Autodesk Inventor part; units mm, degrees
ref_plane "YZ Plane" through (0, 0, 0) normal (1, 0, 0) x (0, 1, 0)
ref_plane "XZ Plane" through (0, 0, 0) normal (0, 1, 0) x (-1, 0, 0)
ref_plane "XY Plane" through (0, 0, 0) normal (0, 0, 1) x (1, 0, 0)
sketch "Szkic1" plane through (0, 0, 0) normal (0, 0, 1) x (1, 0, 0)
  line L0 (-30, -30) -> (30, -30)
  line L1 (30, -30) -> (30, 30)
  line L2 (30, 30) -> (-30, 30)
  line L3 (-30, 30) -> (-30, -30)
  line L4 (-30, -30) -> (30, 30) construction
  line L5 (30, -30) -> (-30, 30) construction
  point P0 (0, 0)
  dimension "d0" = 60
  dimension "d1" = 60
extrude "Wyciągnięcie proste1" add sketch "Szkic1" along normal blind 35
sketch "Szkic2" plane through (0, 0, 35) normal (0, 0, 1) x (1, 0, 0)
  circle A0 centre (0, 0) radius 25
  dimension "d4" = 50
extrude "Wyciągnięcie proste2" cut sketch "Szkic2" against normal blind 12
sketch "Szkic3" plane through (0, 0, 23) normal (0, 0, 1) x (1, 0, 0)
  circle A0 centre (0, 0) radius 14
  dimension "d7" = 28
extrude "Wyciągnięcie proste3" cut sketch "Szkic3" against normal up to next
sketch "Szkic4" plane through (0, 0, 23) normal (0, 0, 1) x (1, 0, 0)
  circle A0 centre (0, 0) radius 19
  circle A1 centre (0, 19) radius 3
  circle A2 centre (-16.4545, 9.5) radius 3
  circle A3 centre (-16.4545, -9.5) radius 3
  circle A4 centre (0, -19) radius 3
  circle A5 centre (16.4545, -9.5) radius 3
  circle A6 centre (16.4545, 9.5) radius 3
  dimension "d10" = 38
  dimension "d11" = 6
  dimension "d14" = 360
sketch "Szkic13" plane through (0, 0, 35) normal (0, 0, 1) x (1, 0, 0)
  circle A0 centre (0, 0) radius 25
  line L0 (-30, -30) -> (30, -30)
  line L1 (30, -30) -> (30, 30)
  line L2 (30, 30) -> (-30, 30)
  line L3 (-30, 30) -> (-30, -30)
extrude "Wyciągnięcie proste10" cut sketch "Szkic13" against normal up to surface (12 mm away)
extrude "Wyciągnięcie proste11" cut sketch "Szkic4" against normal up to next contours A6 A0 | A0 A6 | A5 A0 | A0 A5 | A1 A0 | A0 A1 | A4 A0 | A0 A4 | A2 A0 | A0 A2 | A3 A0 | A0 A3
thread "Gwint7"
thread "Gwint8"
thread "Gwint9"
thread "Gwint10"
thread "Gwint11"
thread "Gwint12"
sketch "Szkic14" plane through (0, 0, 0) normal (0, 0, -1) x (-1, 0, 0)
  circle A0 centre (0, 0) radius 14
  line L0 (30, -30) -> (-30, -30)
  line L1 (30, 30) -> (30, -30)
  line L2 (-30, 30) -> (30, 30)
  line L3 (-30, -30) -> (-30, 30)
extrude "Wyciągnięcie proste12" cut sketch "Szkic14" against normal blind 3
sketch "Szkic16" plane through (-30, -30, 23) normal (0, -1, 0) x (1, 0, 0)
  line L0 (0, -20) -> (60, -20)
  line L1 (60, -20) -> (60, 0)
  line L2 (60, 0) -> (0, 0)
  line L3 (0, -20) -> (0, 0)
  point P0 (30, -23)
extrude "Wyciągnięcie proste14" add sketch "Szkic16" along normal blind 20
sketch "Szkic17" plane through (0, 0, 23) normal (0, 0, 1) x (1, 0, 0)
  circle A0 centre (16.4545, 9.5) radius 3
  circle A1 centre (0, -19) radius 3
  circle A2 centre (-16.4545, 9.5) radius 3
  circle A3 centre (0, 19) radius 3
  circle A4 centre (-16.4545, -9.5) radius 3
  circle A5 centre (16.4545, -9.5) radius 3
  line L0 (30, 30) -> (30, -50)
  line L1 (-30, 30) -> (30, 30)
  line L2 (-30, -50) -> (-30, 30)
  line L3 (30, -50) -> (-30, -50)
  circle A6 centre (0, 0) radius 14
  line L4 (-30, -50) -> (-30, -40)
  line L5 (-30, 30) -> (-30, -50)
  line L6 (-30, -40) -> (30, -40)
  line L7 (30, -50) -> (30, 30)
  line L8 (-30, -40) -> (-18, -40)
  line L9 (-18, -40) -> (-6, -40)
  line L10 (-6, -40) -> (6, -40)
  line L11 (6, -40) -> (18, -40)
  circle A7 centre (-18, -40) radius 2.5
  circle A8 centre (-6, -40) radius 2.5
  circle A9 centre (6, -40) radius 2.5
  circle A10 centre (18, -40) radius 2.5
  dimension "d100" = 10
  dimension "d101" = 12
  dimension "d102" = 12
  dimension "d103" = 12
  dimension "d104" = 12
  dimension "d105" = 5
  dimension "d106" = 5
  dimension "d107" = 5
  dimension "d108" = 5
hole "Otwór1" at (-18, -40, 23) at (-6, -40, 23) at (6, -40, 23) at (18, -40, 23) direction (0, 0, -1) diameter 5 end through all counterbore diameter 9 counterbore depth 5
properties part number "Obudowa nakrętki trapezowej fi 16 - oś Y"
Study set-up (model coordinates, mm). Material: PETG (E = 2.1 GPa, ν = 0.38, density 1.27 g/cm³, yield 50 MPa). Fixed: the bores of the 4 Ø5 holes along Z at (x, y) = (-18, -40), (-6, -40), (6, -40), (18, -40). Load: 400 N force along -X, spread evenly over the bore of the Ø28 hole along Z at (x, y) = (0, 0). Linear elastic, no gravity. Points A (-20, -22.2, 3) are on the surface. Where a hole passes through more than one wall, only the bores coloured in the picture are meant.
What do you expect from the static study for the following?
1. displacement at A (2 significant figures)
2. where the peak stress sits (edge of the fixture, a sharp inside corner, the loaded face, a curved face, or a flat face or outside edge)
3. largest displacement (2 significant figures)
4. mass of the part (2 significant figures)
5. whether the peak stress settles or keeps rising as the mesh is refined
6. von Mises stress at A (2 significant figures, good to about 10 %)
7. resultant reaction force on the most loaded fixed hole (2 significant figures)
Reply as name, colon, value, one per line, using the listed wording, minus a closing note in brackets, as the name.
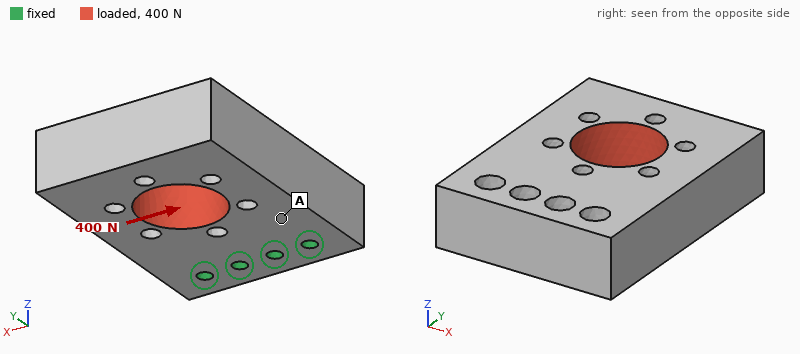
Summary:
displacement at A: 0.021 mm
where the peak stress sits: edge of the fixture
largest displacement: 0.11 mm
mass of the part: 99 g
whether the peak stress settles or keeps rising as the mesh is refined: keeps rising
von Mises stress at A: 0.58 MPa
resultant reaction force on the most loaded fixed hole: 400 N
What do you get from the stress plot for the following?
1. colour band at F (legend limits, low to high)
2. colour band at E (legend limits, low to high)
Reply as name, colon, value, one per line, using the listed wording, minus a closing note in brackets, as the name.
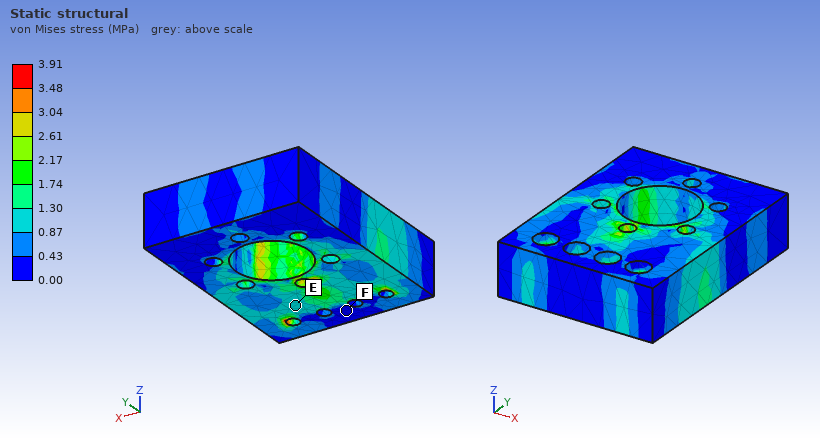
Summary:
colour band at F: 0.00 to 0.43 MPa
colour band at E: 0.87 to 1.30 MPa
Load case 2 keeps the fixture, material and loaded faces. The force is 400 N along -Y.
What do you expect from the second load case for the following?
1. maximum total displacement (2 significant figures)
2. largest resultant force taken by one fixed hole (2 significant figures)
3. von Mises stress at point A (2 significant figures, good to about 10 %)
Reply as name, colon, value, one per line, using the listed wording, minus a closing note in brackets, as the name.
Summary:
maximum total displacement: 24 µm
largest resultant force taken by one fixed hole: 140 N
von Mises stress at point A: 0.38 MPa
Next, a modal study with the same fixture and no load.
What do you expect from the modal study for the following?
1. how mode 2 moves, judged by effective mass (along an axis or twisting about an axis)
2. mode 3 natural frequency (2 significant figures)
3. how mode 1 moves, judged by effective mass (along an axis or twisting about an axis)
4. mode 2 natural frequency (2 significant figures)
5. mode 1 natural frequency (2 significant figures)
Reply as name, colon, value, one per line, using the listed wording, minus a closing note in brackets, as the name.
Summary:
how mode 2 moves, judged by effective mass: along X
mode 3 natural frequency: 1400 Hz
how mode 1 moves, judged by effective mass: along Z
mode 2 natural frequency: 1300 Hz
mode 1 natural frequency: 690 Hz
